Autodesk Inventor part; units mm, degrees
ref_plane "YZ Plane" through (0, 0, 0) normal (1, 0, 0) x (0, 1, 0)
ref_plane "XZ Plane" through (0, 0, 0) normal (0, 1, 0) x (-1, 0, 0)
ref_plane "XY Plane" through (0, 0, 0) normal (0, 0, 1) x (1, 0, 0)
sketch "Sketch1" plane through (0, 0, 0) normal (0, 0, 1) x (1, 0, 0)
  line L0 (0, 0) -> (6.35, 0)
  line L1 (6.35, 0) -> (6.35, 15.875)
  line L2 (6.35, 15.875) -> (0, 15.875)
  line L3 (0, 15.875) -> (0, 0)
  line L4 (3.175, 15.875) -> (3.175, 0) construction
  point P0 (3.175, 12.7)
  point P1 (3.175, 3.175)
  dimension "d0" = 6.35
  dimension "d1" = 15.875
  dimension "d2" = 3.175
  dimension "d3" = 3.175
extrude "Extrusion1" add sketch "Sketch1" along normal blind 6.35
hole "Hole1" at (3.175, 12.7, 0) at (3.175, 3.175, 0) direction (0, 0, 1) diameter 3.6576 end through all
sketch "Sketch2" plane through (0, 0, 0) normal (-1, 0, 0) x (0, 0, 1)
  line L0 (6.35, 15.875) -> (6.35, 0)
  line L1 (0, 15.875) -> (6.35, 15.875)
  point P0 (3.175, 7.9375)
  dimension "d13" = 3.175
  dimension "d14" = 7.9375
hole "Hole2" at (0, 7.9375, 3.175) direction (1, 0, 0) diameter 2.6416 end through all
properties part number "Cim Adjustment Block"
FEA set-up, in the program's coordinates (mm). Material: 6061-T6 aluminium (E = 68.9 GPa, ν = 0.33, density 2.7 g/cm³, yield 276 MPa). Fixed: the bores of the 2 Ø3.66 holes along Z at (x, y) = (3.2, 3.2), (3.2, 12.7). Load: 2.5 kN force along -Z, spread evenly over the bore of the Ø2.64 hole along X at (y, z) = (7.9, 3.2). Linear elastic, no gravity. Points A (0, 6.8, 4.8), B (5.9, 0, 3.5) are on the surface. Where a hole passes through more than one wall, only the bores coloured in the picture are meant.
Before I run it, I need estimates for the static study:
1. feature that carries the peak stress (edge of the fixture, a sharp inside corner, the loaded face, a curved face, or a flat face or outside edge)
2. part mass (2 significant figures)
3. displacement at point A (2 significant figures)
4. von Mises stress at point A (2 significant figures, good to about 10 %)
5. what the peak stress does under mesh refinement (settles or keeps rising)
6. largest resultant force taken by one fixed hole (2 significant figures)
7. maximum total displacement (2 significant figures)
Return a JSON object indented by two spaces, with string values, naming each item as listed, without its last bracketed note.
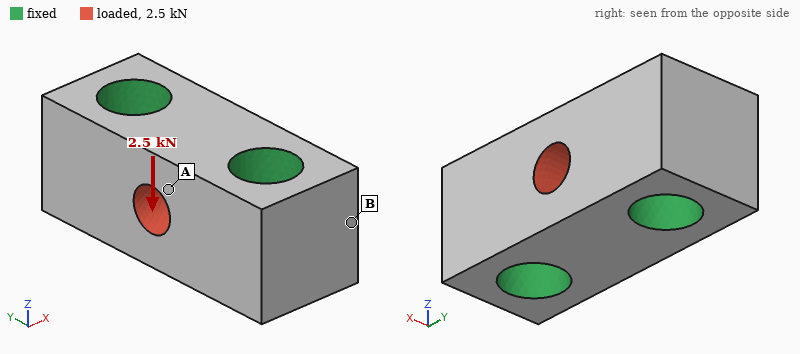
{
  "feature that carries the peak stress": "edge of the fixture",
  "part mass": "1.3 g",
  "displacement at point A": "3.7 µm",
  "von Mises stress at point A": "58 MPa",
  "what the peak stress does under mesh refinement": "keeps rising",
  "largest resultant force taken by one fixed hole": "1.3 kN",
  "maximum total displacement": "5.2 µm"
}
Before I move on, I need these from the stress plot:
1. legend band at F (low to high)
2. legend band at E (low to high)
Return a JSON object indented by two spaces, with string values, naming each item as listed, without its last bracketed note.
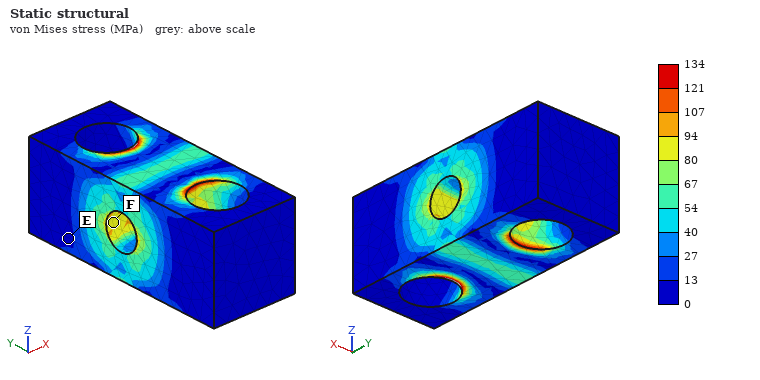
{
  "legend band at F": "80 to 94 MPa",
  "legend band at E": "0 to 13 MPa"
}
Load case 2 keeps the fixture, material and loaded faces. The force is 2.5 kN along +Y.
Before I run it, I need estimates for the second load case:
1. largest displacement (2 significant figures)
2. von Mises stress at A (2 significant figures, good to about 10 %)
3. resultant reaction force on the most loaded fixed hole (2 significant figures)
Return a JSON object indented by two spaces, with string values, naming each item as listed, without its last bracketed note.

{
  "largest displacement": "2.1 µm",
  "von Mises stress at A": "33 MPa",
  "resultant reaction force on the most loaded fixed hole": "1.3 kN"
}
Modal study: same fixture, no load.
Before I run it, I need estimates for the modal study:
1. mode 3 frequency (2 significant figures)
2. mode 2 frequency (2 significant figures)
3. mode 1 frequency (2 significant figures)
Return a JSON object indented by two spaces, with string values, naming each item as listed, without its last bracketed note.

{
  "mode 3 frequency": "220 kHz",
  "mode 2 frequency": "210 kHz",
  "mode 1 frequency": "210 kHz"
}
